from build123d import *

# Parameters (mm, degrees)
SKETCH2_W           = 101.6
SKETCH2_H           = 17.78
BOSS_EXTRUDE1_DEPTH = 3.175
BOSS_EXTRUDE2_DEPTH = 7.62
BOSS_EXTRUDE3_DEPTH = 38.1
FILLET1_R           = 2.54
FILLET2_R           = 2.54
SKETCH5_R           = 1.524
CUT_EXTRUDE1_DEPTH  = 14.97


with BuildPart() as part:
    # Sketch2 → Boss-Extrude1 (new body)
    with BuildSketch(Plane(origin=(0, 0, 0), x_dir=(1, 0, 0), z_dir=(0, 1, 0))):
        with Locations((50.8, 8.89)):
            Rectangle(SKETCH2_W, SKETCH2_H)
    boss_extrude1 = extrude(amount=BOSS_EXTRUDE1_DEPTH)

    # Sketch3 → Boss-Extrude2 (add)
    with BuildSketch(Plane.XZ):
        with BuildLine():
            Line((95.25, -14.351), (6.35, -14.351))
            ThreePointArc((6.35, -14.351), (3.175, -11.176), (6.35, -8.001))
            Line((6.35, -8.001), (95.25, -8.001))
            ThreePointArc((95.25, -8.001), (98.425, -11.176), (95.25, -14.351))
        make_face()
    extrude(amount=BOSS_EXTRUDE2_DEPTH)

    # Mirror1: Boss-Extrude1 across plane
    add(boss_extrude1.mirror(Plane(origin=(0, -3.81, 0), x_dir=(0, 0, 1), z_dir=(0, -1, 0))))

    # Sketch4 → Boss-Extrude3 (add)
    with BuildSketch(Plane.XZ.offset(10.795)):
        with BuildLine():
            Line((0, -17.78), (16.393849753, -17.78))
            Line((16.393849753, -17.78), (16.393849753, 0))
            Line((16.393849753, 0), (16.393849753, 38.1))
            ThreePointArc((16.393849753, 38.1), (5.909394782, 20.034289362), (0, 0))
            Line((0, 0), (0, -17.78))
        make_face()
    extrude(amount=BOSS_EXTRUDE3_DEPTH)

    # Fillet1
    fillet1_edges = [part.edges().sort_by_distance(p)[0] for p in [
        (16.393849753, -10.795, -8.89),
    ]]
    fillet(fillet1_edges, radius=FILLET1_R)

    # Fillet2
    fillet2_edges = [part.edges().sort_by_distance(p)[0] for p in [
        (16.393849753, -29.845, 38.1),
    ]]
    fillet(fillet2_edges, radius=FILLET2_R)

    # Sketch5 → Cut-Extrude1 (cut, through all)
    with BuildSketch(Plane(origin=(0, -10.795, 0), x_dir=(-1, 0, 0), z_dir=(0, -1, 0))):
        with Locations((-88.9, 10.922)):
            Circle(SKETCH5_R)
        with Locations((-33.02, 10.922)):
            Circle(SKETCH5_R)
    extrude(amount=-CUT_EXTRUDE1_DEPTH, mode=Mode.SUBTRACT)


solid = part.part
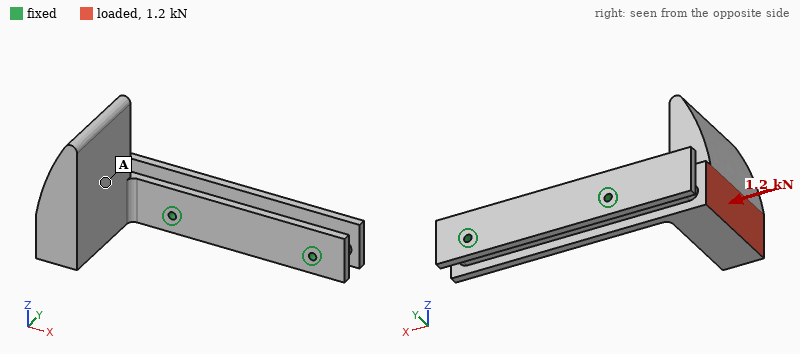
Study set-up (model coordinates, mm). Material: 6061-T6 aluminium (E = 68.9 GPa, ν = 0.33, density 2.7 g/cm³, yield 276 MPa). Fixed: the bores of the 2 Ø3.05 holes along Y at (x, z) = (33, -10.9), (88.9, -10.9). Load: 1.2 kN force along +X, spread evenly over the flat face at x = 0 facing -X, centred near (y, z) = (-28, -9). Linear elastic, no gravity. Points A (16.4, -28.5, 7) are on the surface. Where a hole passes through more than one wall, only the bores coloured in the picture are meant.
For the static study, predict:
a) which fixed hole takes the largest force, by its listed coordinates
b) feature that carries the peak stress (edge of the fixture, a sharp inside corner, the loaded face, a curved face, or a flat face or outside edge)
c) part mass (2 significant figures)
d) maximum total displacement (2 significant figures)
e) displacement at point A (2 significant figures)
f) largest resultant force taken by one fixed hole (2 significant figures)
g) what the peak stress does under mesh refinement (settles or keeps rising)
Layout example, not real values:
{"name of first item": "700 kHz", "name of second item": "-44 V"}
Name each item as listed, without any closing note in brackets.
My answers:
{"which fixed hole takes the largest force, by its listed coordinates": "(33, -10.9)", "feature that carries the peak stress": "edge of the fixture", "part mass": "110 g", "maximum total displacement": "0.23 mm", "displacement at point A": "0.11 mm", "largest resultant force taken by one fixed hole": "1.1 kN", "what the peak stress does under mesh refinement": "keeps rising"}
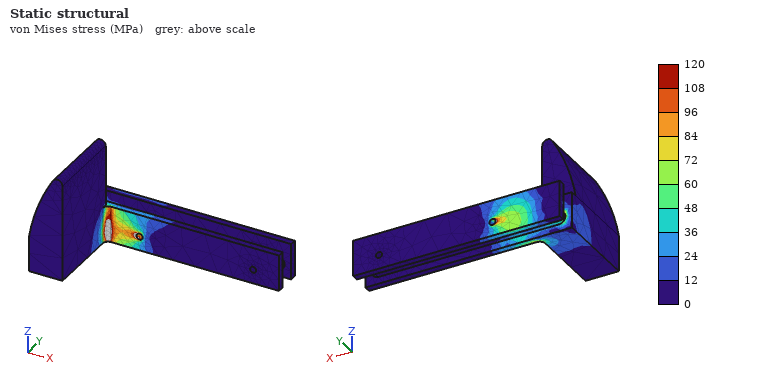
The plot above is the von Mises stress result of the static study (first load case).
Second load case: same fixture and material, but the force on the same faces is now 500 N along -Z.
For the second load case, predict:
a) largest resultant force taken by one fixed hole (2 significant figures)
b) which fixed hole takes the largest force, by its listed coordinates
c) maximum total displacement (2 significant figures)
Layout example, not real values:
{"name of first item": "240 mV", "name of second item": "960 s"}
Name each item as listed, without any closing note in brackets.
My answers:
{"largest resultant force taken by one fixed hole": "740 N", "which fixed hole takes the largest force, by its listed coordinates": "(33, -10.9)", "maximum total displacement": "0.42 mm"}
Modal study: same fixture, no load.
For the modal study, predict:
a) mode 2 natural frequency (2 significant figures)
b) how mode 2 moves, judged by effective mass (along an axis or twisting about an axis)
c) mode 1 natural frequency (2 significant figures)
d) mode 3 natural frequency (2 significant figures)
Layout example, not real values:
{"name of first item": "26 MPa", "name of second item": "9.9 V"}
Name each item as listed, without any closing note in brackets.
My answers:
{"mode 2 natural frequency": "1400 Hz", "how mode 2 moves, judged by effective mass": "along X", "mode 1 natural frequency": "760 Hz", "mode 3 natural frequency": "2800 Hz"}
